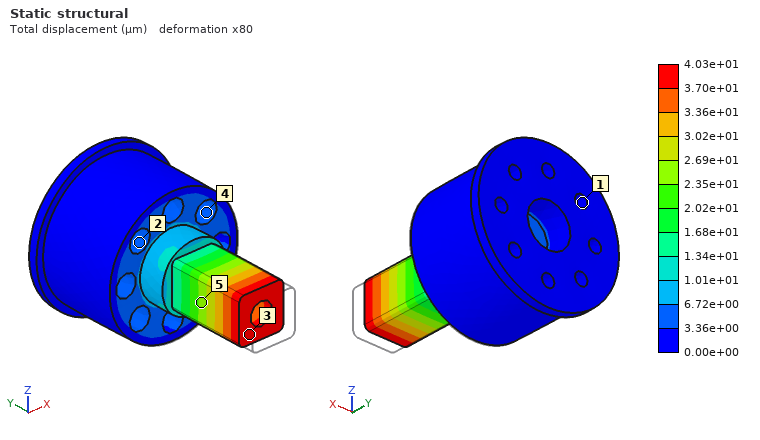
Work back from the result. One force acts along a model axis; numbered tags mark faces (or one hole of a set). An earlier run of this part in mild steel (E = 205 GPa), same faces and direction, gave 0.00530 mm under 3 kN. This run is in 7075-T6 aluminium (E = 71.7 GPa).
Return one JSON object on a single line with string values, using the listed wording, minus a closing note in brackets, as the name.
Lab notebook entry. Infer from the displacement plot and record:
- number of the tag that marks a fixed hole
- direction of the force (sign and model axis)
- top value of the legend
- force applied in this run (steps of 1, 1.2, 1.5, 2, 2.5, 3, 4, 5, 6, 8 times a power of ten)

{"number of the tag that marks a fixed hole": "1", "direction of the force": "+Y", "top value of the legend": "4.03e+01 µm", "force applied in this run": "8 kN"}
